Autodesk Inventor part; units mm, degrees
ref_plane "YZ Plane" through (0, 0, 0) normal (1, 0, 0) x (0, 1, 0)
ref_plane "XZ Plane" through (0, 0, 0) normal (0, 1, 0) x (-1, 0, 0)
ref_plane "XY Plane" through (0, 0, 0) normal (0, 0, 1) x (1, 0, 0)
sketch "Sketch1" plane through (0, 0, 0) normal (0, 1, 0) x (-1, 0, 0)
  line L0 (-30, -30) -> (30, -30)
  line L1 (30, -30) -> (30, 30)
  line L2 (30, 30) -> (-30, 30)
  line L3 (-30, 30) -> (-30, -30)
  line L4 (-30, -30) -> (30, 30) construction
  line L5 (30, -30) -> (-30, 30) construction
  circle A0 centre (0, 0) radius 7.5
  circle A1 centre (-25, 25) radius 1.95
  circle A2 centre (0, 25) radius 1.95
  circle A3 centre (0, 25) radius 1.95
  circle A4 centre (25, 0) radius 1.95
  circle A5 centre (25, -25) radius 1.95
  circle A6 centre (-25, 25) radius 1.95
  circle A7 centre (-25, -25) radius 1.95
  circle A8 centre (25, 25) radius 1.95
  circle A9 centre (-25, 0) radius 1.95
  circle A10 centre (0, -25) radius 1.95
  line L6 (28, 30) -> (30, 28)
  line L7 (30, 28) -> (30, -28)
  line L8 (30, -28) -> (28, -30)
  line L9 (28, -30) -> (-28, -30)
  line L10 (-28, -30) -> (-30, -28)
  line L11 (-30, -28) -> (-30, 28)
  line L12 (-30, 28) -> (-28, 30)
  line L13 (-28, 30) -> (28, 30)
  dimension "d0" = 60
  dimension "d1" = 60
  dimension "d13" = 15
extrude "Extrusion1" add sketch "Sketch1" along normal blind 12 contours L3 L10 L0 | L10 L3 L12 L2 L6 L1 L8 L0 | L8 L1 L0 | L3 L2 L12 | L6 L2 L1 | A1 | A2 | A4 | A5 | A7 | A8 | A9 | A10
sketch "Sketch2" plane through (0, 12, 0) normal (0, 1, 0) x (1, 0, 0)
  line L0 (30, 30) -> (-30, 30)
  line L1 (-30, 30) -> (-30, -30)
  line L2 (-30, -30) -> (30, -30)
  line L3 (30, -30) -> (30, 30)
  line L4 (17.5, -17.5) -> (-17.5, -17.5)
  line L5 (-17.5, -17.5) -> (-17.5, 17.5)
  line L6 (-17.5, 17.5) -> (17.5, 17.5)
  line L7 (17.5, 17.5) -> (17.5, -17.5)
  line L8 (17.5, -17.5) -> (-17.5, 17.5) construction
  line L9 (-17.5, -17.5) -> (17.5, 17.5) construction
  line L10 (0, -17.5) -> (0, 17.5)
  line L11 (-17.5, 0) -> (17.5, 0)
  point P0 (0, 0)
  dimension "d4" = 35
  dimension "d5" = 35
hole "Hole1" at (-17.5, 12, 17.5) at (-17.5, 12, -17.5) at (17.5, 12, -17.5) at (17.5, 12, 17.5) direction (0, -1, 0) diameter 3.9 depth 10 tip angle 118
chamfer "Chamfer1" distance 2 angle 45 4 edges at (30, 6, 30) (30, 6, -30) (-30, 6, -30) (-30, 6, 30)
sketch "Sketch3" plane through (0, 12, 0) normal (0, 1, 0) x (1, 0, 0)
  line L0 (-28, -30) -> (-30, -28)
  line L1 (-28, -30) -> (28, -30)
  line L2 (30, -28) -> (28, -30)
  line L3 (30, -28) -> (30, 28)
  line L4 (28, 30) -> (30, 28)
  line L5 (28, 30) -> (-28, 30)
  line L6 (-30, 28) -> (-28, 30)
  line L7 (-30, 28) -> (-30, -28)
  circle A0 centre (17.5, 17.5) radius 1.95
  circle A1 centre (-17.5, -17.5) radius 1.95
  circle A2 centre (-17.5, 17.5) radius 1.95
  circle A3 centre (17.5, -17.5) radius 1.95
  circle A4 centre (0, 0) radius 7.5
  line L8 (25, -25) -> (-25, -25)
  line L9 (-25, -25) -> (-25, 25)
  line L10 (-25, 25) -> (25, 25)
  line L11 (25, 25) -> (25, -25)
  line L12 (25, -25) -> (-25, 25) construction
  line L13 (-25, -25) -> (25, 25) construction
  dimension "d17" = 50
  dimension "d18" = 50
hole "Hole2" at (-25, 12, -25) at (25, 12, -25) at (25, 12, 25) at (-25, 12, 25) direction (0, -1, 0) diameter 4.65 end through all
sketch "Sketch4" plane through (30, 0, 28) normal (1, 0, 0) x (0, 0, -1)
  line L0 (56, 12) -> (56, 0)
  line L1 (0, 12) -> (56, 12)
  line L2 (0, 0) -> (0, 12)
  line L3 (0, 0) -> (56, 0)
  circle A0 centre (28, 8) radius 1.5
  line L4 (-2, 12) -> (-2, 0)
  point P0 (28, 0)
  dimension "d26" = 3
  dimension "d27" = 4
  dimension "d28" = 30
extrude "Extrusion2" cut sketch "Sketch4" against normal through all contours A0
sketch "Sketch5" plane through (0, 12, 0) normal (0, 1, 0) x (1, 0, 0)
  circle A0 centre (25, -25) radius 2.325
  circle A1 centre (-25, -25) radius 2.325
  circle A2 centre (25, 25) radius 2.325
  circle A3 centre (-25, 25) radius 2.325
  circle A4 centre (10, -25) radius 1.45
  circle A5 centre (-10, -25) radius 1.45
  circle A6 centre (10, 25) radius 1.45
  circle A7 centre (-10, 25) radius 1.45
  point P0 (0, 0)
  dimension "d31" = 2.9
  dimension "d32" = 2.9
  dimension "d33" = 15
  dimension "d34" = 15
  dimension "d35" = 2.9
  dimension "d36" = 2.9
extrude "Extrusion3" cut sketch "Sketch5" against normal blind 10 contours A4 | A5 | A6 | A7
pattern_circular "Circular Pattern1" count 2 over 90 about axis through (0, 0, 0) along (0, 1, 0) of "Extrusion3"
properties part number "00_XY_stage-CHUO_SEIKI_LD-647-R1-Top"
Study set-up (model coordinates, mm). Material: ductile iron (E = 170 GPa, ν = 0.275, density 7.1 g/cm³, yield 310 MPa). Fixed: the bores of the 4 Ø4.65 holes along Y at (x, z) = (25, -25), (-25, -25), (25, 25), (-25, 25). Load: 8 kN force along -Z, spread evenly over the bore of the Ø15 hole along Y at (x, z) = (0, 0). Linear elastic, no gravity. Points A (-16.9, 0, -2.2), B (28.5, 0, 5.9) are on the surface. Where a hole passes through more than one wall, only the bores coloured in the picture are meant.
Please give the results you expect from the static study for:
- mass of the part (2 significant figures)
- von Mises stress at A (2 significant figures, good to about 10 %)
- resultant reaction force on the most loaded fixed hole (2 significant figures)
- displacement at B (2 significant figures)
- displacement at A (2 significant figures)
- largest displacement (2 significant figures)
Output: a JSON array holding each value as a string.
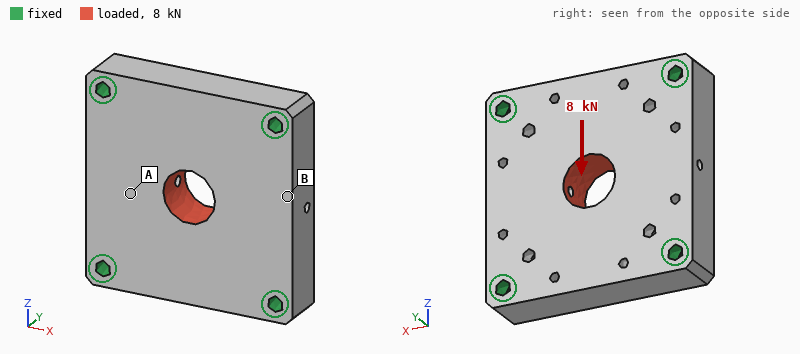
["280 g", "10 MPa", "2.2 kN", "0.73 µm", "1.5 µm", "3.1 µm"]
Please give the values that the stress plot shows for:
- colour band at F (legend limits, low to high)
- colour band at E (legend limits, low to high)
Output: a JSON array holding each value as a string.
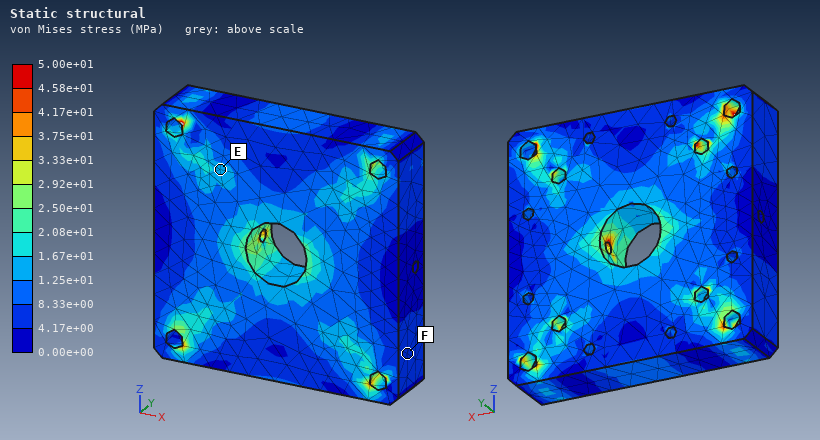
["4.17e+00 to 8.33e+00 MPa", "1.25e+01 to 1.67e+01 MPa"]
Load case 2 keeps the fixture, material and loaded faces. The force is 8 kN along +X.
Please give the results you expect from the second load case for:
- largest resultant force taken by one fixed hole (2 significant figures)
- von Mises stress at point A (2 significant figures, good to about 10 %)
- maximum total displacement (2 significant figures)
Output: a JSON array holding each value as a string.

["2.2 kN", "6.8 MPa", "3.1 µm"]
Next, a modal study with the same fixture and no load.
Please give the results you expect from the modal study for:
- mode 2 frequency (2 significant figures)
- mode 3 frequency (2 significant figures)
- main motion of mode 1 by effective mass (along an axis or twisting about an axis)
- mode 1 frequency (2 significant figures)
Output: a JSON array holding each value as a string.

["19 kHz", "20 kHz", "along Y", "13 kHz"]
